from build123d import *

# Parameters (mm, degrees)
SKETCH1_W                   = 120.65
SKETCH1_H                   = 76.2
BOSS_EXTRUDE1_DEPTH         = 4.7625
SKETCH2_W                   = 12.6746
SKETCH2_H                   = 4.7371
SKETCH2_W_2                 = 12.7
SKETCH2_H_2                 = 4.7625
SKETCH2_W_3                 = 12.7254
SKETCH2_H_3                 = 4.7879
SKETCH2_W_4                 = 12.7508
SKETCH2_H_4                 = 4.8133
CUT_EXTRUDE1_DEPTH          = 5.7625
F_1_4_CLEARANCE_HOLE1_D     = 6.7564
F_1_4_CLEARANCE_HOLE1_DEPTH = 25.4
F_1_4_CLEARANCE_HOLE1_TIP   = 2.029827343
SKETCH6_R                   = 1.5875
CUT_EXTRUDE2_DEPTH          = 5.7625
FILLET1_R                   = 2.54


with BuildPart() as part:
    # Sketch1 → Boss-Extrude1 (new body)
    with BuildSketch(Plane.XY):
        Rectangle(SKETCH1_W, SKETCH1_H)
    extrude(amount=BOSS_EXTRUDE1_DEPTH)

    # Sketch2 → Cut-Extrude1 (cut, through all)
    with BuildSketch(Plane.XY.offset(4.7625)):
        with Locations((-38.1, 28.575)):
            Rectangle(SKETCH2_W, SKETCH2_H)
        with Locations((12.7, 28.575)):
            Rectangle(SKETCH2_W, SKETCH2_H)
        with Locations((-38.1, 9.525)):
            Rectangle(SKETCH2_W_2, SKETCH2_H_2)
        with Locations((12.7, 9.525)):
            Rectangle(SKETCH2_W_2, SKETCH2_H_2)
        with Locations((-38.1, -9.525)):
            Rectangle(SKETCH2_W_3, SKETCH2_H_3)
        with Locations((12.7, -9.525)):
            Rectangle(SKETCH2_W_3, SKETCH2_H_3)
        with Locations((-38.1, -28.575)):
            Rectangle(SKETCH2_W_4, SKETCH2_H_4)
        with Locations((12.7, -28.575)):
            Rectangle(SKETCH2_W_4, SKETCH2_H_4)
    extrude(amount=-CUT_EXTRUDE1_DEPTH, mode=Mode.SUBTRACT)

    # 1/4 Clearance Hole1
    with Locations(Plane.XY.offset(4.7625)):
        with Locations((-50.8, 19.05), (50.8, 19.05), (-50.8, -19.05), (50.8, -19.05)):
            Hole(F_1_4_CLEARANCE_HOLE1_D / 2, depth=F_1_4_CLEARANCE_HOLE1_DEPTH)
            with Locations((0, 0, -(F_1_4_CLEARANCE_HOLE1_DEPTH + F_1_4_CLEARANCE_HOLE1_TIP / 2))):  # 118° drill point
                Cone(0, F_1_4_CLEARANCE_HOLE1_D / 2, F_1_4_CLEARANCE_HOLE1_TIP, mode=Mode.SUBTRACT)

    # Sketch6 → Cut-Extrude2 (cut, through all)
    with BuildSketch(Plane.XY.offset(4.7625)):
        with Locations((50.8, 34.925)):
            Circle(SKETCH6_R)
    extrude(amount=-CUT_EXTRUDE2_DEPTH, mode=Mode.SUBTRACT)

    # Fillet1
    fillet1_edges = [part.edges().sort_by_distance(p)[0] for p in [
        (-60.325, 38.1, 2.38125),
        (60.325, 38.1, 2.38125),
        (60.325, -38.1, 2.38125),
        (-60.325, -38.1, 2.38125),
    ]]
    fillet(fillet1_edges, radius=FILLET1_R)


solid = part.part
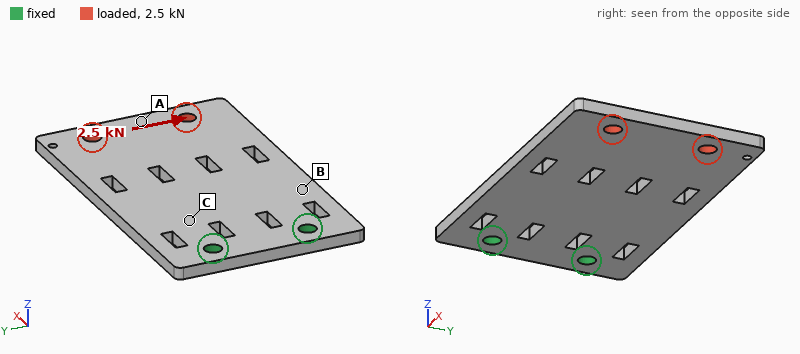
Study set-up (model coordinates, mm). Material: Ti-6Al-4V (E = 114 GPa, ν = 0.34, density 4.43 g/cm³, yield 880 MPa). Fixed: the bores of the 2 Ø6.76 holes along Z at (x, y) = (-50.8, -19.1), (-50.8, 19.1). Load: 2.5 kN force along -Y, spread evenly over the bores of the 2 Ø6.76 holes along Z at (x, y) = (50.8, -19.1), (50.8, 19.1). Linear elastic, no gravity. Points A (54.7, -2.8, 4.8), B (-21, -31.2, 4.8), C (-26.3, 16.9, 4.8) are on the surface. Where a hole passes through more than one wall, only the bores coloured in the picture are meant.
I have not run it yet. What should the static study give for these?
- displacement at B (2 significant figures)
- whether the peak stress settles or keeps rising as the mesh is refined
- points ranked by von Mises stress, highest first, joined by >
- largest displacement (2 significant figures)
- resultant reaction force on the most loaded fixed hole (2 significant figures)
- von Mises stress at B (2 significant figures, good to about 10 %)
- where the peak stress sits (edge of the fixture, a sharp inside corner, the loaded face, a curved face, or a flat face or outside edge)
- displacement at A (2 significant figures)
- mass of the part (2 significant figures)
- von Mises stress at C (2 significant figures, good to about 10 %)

0.037 mm
keeps rising
C > B > A
0.13 mm
5.9 kN
25 MPa
edge of the fixture
0.12 mm
180 g
42 MPa
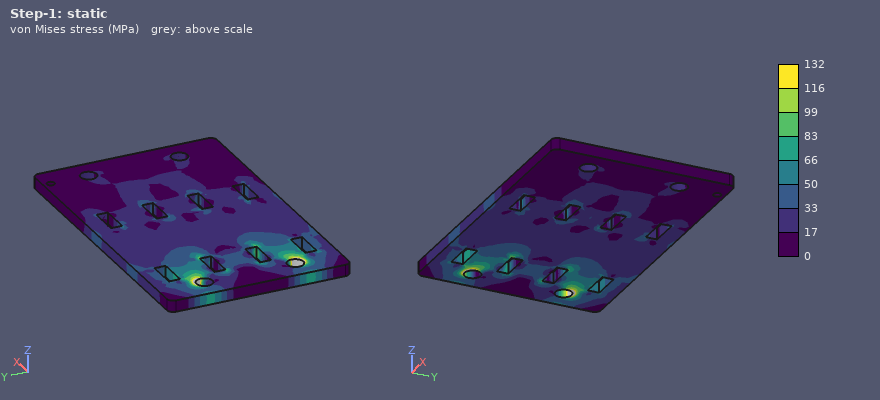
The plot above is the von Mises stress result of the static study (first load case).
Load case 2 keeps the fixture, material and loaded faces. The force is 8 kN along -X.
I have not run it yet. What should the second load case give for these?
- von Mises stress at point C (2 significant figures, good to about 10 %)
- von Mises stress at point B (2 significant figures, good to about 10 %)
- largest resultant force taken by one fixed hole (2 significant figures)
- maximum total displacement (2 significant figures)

32 MPa
18 MPa
4.0 kN
30 µm
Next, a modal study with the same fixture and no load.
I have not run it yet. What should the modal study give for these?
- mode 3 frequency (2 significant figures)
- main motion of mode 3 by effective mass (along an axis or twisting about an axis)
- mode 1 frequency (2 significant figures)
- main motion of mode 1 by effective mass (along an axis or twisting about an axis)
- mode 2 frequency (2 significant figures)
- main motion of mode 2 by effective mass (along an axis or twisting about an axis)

1900 Hz
along Z
300 Hz
along Z
970 Hz
twisting about X
